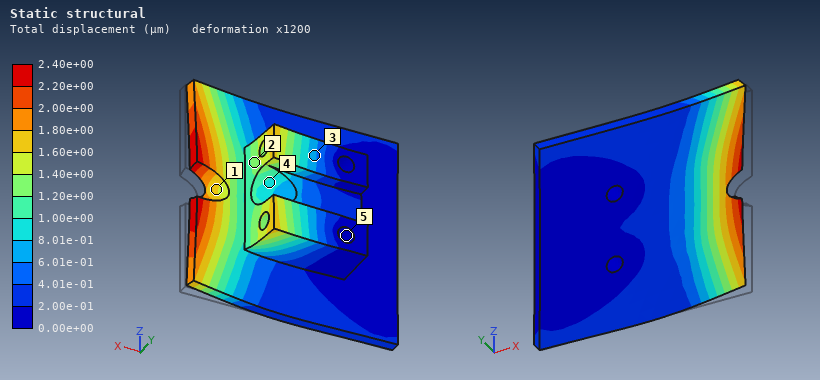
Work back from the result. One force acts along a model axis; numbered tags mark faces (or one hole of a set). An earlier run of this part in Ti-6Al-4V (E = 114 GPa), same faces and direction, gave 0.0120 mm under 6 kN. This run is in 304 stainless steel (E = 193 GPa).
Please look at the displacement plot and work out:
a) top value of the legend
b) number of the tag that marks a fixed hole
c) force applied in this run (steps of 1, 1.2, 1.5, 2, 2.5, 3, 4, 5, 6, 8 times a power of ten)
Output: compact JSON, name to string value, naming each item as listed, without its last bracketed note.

{"top value of the legend": "2.40e+00 µm", "number of the tag that marks a fixed hole": "5", "force applied in this run": "2 kN"}
